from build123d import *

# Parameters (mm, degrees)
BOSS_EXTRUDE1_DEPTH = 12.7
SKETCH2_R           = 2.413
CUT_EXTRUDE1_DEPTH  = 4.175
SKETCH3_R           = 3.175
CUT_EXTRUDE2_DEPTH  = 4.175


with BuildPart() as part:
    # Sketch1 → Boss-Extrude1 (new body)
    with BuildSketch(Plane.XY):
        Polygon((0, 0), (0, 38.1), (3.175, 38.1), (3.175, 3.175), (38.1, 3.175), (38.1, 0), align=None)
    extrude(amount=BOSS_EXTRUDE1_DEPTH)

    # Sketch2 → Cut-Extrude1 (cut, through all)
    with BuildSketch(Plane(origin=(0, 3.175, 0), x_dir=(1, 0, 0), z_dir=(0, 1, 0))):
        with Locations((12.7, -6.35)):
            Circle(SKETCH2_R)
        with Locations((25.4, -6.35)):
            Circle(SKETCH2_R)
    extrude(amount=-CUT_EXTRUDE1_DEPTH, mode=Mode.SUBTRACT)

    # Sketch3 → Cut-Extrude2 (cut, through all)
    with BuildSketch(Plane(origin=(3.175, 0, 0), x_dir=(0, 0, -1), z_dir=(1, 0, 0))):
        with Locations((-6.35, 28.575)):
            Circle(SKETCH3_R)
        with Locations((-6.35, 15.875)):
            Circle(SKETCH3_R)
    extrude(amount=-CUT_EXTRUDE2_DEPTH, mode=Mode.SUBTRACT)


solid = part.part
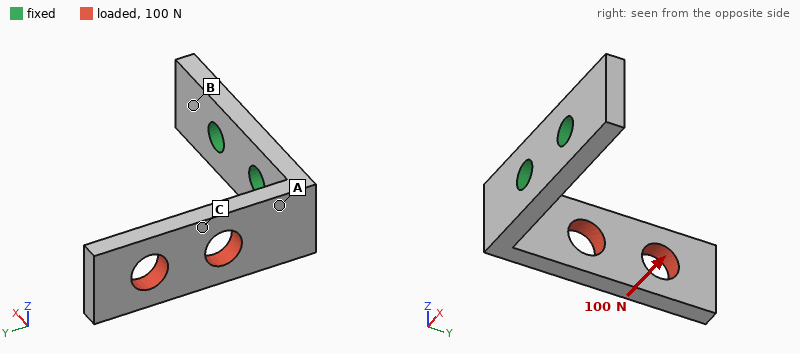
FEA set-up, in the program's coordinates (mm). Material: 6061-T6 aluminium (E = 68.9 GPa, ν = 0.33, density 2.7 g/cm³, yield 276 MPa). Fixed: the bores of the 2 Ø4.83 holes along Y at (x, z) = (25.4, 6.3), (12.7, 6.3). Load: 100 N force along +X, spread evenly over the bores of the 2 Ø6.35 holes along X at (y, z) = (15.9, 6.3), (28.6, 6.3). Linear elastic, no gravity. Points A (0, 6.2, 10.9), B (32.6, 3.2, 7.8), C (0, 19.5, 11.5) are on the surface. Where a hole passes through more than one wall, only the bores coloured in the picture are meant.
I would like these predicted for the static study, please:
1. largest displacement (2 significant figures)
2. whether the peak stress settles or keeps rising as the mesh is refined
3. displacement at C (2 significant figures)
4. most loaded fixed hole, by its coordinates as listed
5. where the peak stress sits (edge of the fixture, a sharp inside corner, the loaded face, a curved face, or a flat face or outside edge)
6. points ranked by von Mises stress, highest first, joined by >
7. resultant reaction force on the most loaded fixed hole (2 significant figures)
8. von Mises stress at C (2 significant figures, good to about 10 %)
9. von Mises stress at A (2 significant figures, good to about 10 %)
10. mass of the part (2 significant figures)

0.60 mm
keeps rising
0.25 mm
(12.7, 6.3)
edge of the fixture
A > C > B
93 N
33 MPa
74 MPa
7.1 g
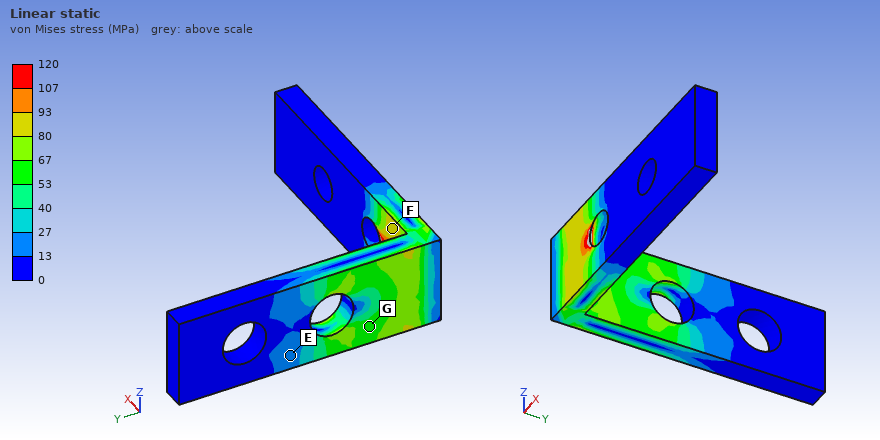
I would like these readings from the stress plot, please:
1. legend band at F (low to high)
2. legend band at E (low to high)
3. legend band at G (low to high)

80 to 93 MPa
13 to 27 MPa
53 to 67 MPa
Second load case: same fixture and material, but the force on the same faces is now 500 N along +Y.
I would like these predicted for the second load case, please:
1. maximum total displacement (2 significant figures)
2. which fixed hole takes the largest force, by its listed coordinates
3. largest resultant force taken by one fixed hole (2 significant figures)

0.37 mm
(12.7, 6.3)
530 N
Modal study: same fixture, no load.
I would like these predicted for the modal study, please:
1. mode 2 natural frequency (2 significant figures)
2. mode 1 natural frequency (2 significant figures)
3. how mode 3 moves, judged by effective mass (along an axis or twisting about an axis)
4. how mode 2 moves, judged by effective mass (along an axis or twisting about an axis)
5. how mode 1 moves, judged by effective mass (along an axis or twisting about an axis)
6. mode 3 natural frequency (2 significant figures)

2500 Hz
1400 Hz
along Y
along Z
along X
7100 Hz
